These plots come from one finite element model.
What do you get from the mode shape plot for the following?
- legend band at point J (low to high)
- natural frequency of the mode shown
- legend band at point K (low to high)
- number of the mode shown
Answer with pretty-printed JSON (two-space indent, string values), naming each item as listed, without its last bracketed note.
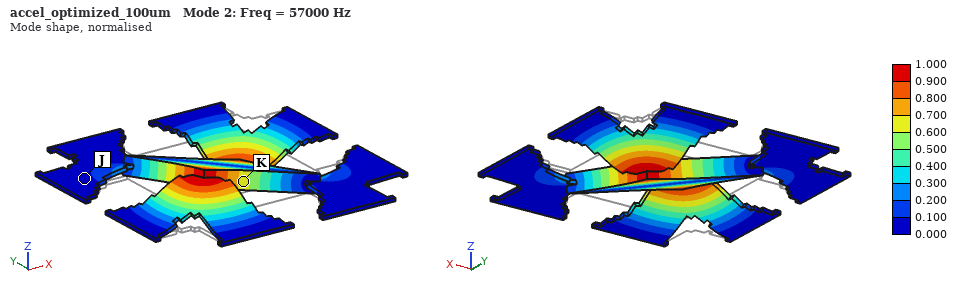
{
  "legend band at point J": "0.000 to 0.100",
  "natural frequency of the mode shown": "57000 Hz",
  "legend band at point K": "0.600 to 0.700",
  "number of the mode shown": "2"
}
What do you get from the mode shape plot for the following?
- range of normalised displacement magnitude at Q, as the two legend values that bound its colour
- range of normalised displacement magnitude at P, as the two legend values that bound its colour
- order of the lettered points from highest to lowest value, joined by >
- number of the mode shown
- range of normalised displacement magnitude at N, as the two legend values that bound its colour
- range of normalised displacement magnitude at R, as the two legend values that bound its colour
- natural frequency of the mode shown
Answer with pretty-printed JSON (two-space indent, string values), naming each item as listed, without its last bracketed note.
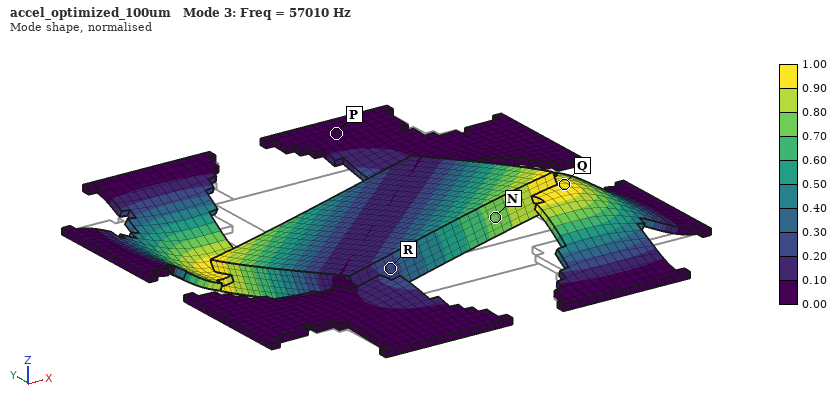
{
  "range of normalised displacement magnitude at Q, as the two legend values that bound its colour": "0.90 to 1.00",
  "range of normalised displacement magnitude at P, as the two legend values that bound its colour": "0.00 to 0.10",
  "order of the lettered points from highest to lowest value, joined by >": "Q > N > R > P",
  "number of the mode shown": "3",
  "range of normalised displacement magnitude at N, as the two legend values that bound its colour": "0.70 to 0.80",
  "range of normalised displacement magnitude at R, as the two legend values that bound its colour": "0.20 to 0.30",
  "natural frequency of the mode shown": "57010 Hz"
}
